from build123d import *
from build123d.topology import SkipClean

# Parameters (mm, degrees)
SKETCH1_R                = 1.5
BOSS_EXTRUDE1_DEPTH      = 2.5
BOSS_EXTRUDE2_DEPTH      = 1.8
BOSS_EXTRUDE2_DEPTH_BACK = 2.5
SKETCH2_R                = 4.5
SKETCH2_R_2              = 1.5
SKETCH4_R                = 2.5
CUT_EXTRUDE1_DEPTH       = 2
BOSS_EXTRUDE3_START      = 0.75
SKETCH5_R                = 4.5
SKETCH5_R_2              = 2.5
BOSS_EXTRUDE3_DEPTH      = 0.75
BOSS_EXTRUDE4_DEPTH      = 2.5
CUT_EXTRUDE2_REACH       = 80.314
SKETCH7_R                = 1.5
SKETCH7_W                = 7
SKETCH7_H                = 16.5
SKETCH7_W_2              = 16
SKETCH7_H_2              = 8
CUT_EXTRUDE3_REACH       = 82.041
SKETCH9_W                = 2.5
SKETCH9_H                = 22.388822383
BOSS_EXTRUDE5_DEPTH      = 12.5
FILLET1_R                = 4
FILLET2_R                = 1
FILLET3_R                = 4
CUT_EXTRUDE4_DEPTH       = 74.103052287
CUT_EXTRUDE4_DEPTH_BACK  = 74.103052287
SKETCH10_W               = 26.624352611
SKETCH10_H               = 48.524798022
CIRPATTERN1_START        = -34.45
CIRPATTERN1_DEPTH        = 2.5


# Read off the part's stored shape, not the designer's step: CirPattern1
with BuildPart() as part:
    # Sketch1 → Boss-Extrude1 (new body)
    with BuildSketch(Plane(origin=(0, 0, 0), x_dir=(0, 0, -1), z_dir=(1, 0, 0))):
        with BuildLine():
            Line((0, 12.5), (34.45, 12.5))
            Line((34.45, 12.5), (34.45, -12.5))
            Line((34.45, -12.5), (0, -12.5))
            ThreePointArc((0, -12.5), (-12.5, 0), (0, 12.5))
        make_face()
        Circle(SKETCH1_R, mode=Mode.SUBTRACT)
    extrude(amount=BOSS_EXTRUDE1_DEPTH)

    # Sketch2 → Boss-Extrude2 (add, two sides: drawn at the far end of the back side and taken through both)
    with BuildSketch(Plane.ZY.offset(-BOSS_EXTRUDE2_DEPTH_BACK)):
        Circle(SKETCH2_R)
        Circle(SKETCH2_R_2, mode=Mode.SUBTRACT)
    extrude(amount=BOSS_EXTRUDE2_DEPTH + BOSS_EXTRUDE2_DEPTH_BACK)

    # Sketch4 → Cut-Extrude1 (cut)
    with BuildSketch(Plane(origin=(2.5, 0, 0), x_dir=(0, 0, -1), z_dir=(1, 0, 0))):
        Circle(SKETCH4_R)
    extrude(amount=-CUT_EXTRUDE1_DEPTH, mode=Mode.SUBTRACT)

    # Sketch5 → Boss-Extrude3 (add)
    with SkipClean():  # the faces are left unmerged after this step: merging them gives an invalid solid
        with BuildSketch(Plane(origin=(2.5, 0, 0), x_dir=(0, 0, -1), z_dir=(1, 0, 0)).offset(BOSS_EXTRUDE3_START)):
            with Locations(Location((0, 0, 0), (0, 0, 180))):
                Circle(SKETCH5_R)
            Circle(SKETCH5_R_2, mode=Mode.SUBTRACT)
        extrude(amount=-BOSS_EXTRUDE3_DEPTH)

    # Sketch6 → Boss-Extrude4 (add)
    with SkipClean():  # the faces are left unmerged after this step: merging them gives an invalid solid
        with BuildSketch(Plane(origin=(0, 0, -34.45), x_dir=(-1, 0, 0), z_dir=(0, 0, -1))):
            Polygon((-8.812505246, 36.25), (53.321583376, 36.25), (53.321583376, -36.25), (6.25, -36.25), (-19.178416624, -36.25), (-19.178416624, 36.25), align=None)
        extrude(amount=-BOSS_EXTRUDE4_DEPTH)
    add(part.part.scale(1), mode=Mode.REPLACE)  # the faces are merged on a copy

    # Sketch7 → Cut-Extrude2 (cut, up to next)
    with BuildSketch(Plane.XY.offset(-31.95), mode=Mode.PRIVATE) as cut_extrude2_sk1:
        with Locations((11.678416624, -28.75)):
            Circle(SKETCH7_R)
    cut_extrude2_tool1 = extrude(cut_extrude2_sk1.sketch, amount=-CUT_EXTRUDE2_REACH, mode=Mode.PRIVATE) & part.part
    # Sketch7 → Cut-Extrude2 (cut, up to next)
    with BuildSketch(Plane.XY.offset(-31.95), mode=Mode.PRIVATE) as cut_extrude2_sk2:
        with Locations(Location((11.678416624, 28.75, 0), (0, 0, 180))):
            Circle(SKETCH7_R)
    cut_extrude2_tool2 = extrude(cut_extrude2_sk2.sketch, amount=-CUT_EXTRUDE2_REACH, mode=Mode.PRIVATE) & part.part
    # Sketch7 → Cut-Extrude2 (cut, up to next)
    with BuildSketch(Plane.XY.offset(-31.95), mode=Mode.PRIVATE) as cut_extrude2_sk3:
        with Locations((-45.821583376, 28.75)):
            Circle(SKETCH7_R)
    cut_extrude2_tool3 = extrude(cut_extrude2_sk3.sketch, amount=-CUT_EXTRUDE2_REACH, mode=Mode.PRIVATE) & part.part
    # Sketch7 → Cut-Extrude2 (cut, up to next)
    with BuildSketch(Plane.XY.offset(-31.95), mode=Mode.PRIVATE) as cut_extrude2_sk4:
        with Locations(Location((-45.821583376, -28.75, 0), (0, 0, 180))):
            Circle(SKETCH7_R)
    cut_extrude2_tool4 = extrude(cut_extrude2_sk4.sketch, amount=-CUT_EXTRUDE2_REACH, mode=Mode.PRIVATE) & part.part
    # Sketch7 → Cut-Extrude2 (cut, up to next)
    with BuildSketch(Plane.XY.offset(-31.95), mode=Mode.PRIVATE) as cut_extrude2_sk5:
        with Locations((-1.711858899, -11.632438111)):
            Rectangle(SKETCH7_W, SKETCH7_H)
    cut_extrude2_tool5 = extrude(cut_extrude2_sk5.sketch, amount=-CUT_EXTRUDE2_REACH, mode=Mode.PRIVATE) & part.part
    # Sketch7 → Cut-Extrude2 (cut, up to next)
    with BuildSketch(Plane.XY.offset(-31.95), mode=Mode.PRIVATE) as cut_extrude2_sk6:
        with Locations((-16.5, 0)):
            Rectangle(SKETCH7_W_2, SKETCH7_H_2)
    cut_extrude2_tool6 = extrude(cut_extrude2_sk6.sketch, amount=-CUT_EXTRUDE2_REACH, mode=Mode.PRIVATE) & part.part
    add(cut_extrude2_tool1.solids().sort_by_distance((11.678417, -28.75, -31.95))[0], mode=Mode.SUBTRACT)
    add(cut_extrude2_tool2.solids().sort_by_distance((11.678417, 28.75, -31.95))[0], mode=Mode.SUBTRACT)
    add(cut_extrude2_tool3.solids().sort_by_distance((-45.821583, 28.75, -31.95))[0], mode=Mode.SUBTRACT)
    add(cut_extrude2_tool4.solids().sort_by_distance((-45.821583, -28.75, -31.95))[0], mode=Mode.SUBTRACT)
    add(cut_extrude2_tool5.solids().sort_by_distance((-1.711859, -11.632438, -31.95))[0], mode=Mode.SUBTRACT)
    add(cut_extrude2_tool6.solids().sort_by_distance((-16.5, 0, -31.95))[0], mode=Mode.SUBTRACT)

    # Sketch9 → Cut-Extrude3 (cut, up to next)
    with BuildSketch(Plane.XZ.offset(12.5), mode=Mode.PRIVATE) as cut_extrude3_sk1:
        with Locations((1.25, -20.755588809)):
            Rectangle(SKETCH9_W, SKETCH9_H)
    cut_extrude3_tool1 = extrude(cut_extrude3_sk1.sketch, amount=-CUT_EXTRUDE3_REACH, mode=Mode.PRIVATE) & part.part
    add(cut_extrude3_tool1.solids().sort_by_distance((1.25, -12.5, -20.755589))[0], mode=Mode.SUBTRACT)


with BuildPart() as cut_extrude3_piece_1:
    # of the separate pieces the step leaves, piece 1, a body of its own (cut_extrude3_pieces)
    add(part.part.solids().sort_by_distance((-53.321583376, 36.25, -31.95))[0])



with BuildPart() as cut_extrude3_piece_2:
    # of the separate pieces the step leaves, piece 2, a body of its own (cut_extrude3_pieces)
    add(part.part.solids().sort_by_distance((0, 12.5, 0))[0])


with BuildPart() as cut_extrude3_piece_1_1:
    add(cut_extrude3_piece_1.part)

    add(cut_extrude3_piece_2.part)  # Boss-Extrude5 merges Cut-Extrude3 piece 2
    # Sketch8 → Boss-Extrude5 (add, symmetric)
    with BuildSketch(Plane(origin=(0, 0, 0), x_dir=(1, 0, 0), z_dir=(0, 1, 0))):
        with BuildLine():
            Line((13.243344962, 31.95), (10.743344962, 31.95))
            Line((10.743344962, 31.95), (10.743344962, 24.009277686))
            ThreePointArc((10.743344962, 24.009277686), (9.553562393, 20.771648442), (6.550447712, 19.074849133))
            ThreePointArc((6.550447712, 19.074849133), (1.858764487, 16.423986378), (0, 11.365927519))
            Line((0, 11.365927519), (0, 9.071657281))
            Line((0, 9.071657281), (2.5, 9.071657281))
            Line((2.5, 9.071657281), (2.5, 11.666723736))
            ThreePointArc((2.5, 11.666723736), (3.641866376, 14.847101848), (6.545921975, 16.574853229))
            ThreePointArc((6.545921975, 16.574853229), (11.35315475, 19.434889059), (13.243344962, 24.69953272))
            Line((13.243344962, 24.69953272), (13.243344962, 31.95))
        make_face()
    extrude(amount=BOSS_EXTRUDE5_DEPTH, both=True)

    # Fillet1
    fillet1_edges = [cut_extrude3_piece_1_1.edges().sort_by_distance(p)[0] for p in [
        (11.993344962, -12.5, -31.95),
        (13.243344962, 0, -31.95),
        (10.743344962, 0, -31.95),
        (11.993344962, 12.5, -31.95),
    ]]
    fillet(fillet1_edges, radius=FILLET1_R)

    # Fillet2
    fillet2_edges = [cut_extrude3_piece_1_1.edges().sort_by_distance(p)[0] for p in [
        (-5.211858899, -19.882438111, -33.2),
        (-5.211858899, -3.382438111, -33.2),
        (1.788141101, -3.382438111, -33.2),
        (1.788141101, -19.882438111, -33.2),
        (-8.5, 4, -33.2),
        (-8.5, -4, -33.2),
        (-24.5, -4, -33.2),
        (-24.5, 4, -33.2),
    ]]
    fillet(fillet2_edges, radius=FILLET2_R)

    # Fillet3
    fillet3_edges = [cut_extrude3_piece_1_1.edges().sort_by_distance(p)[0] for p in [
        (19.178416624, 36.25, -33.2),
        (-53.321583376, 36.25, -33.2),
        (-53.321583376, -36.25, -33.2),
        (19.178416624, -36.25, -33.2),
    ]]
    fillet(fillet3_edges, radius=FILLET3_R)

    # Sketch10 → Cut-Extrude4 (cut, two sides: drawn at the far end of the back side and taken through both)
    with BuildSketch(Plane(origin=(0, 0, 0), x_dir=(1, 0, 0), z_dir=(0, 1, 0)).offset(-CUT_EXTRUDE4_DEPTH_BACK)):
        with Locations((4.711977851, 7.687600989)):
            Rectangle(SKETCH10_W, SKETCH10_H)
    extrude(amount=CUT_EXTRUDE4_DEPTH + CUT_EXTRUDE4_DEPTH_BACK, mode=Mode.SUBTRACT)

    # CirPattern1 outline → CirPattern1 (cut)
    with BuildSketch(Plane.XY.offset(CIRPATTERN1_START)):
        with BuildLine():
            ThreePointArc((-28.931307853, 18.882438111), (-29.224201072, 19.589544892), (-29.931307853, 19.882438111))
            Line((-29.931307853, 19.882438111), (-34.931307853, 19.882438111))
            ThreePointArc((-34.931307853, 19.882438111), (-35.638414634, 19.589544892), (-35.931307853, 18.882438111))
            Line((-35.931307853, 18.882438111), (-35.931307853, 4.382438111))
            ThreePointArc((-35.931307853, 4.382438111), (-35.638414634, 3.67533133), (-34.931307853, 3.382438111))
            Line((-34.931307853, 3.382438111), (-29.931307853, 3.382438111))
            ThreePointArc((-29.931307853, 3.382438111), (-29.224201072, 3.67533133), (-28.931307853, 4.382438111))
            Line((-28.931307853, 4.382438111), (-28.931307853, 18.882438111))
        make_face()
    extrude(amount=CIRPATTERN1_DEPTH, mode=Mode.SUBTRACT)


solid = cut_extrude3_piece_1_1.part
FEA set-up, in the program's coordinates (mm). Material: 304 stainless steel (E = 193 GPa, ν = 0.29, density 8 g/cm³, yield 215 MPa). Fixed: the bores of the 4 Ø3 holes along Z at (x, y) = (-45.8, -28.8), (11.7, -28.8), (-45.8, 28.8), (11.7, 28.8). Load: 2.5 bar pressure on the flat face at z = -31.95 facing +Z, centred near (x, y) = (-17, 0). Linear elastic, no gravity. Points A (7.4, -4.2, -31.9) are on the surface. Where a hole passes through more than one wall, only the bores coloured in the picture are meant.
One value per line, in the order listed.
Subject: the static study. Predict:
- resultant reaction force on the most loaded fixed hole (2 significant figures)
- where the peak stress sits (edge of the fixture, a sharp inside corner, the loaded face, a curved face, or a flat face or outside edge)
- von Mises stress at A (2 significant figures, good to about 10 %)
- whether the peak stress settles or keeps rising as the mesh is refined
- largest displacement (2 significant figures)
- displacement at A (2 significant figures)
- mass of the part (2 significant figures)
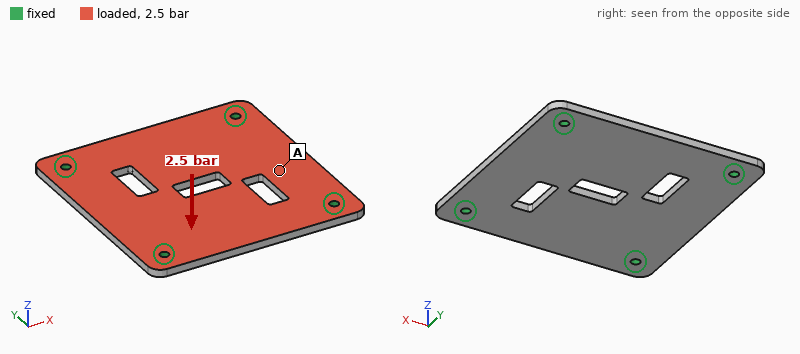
310 N
edge of the fixture
46 MPa
keeps rising
84 µm
47 µm
97 g
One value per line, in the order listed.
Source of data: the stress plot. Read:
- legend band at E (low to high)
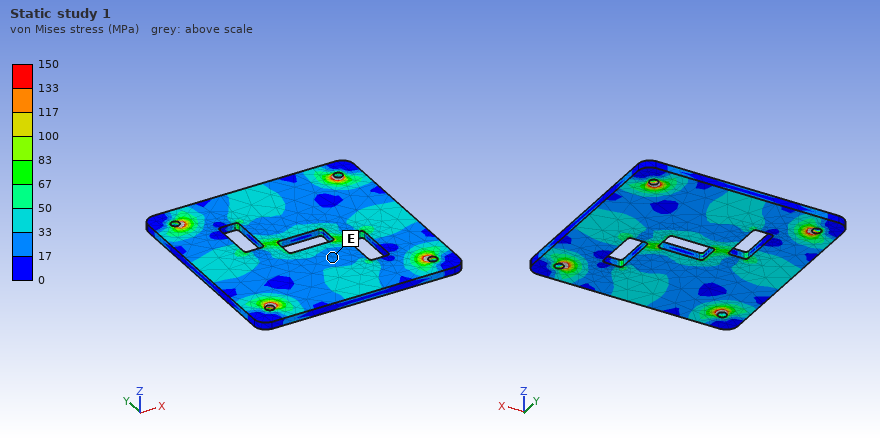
17 to 33 MPa
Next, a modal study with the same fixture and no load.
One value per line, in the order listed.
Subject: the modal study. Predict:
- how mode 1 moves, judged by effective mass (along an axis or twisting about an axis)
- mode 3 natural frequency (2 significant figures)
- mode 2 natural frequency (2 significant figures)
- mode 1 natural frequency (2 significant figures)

along Z
4100 Hz
4000 Hz
2500 Hz
